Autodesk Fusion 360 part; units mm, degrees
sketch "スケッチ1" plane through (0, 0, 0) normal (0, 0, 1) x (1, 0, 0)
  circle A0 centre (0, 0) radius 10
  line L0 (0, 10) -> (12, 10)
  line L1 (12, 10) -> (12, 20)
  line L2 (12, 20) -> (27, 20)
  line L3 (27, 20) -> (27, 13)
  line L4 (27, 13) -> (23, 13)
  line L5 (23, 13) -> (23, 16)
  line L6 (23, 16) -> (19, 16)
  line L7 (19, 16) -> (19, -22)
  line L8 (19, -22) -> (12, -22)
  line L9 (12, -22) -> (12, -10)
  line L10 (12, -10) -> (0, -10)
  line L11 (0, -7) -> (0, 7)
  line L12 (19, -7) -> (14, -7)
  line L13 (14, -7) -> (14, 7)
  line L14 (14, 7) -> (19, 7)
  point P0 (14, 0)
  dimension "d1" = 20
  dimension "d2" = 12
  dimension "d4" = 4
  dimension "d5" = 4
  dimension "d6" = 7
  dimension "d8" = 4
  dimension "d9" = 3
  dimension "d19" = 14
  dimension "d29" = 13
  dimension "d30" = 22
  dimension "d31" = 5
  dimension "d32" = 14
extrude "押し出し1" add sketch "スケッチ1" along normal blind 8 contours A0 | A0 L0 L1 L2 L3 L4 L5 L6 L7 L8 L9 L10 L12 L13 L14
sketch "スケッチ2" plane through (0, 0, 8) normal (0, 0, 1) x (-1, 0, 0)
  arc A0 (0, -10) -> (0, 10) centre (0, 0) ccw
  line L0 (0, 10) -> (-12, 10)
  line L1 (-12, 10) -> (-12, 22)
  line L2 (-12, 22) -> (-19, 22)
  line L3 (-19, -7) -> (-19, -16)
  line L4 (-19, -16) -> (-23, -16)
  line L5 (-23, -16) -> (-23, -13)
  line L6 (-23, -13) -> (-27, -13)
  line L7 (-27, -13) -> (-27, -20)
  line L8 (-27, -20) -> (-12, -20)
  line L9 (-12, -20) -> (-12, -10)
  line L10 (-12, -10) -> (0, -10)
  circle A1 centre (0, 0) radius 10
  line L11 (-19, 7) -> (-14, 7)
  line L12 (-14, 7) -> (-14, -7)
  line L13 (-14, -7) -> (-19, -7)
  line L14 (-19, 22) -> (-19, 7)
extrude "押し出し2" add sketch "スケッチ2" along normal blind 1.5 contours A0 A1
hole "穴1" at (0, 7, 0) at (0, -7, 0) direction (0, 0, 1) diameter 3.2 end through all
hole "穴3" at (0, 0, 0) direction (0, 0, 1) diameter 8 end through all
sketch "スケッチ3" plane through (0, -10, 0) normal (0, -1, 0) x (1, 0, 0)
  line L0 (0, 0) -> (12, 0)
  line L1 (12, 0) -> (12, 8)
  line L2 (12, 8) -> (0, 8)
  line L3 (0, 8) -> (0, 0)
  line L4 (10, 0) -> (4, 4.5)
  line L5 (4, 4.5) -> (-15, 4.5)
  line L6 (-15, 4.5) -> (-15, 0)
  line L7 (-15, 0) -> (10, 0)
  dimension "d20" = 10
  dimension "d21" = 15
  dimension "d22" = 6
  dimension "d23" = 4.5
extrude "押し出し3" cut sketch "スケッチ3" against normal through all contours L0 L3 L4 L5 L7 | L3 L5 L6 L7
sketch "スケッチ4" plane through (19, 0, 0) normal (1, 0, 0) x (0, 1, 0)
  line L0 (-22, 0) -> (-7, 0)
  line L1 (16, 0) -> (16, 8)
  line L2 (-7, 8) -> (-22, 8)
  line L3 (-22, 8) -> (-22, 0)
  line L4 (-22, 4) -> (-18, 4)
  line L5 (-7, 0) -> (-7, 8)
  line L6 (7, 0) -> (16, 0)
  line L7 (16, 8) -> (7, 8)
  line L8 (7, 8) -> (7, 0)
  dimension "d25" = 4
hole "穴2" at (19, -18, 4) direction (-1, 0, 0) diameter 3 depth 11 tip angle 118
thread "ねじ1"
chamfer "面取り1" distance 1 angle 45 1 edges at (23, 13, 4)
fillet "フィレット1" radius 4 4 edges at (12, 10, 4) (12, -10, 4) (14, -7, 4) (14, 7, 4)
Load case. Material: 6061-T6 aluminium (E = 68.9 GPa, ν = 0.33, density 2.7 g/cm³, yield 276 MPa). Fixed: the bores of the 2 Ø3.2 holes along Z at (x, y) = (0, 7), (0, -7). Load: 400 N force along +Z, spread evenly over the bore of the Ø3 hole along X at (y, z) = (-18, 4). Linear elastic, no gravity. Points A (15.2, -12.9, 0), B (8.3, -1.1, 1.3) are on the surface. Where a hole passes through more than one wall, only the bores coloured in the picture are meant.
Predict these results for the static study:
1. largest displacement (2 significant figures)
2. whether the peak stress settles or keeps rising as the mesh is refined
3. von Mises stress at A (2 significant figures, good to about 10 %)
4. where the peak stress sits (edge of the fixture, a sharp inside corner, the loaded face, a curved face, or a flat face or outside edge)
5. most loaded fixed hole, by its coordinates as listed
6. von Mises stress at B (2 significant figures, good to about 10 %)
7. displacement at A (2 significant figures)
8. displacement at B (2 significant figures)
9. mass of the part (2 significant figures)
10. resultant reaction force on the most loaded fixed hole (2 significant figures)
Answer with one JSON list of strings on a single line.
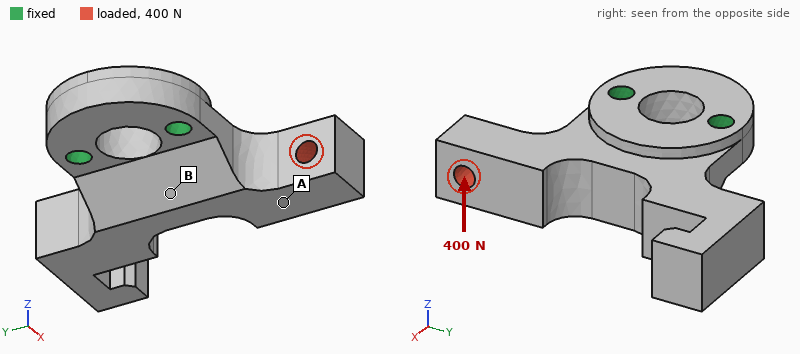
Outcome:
["0.14 mm", "keeps rising", "26 MPa", "edge of the fixture", "(0, -7)", "56 MPa", "0.085 mm", "0.025 mm", "11 g", "630 N"]
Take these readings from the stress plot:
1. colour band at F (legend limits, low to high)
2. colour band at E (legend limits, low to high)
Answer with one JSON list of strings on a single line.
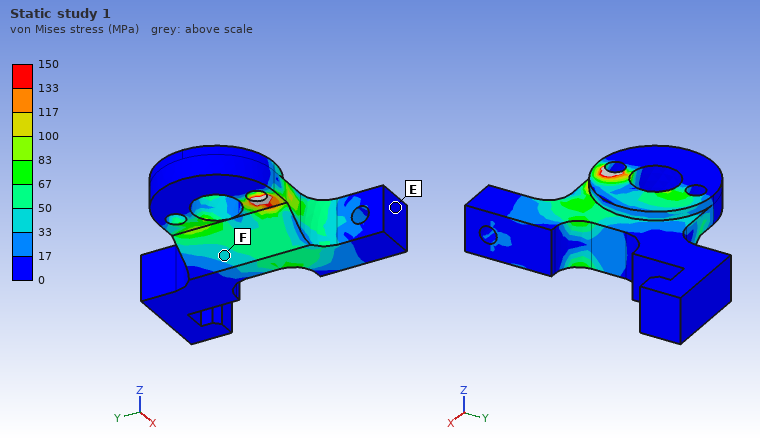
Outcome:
["33 to 50 MPa", "0 to 17 MPa"]
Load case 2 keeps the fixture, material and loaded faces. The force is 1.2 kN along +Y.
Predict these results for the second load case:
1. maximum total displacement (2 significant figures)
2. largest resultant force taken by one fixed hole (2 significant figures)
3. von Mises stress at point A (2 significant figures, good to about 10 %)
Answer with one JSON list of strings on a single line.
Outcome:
["55 µm", "1.4 kN", "26 MPa"]
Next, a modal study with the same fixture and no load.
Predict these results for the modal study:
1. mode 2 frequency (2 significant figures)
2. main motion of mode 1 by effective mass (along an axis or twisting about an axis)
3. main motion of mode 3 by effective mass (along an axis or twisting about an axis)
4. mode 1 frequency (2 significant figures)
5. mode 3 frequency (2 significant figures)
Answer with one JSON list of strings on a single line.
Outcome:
["7600 Hz", "along Z", "along Y", "4900 Hz", "9700 Hz"]
